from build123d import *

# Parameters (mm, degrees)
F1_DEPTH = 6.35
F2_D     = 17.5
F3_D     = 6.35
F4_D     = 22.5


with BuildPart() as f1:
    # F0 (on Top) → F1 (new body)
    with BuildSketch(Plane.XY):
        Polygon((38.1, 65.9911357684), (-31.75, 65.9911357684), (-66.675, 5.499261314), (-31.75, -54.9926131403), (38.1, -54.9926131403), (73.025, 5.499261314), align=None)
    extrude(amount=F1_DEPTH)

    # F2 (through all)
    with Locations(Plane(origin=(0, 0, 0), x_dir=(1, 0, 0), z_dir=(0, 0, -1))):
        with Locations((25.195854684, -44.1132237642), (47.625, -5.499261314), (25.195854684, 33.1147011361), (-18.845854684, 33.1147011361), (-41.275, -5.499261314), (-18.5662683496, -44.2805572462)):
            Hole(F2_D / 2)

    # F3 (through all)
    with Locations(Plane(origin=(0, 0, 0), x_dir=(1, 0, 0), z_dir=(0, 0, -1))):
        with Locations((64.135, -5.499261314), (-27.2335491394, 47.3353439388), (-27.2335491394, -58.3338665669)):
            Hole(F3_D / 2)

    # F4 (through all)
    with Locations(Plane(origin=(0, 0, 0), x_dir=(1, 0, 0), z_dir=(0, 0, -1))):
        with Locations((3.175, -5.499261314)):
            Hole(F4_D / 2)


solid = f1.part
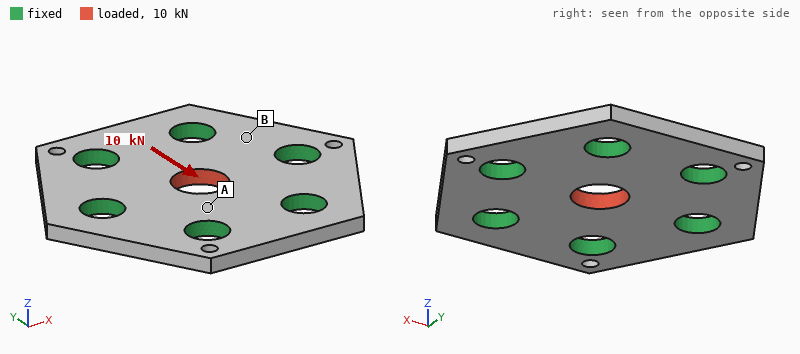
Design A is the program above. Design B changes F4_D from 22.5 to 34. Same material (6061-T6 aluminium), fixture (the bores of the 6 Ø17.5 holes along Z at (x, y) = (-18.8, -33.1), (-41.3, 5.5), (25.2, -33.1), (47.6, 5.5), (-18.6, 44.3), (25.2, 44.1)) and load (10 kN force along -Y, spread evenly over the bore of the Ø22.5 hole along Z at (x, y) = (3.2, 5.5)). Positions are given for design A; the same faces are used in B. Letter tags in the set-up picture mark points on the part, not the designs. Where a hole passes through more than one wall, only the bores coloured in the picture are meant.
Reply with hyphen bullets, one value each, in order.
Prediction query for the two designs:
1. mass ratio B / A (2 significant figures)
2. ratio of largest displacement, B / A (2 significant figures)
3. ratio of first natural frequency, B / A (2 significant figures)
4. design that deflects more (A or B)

- 0.95
- 0.71
- 1.3
- A
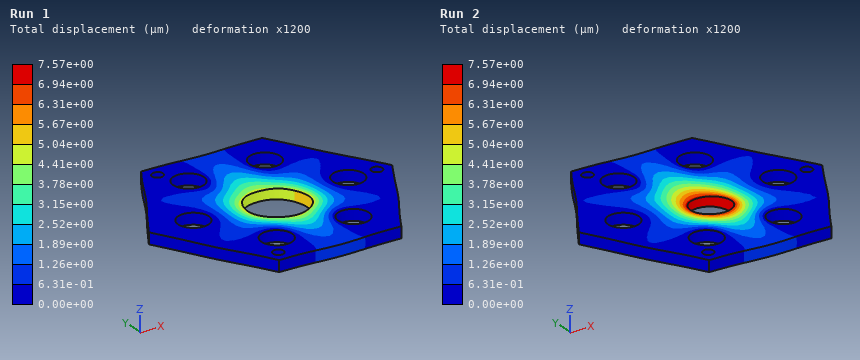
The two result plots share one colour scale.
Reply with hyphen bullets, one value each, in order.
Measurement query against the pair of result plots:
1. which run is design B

- Run 1
